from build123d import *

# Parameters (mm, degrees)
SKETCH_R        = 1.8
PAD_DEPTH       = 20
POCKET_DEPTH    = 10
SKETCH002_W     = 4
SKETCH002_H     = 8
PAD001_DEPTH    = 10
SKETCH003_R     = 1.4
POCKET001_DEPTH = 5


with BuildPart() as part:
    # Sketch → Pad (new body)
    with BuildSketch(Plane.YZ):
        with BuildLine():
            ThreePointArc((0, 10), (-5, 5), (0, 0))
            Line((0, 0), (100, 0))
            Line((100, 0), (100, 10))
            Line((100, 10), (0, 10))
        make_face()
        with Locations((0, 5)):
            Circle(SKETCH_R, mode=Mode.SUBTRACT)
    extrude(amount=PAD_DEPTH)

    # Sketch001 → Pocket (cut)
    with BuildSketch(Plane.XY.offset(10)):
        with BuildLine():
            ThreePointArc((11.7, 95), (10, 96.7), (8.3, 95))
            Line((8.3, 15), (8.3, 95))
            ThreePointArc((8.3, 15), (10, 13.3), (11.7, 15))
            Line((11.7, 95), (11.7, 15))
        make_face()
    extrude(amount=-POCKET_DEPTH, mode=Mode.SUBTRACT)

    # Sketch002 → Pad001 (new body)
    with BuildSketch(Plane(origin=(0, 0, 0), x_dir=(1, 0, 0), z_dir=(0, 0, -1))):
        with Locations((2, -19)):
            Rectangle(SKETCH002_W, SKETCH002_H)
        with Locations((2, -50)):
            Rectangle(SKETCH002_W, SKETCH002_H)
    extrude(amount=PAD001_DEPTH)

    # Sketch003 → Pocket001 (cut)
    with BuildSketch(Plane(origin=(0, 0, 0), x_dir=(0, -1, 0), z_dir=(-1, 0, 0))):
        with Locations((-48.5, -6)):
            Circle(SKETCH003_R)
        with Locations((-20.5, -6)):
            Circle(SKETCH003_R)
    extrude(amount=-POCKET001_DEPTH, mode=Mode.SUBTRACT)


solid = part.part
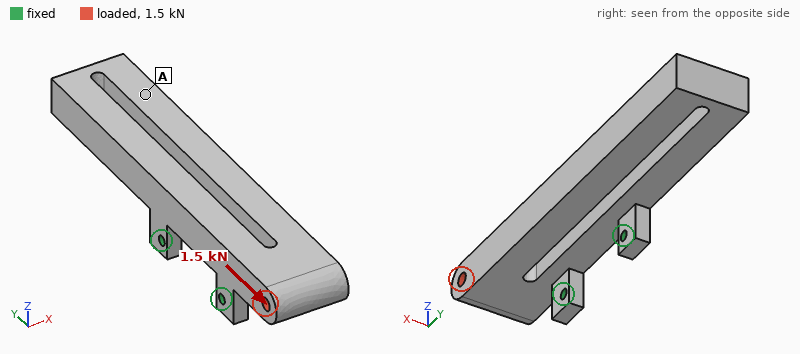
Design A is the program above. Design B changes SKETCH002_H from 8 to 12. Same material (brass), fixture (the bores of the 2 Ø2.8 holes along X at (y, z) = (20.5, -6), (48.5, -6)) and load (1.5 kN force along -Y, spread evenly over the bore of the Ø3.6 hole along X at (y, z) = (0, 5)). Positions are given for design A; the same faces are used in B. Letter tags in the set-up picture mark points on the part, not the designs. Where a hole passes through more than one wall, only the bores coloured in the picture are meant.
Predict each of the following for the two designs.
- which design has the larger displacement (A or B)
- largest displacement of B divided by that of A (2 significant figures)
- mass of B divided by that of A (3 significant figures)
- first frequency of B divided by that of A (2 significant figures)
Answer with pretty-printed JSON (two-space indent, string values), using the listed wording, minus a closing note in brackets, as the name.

{
  "which design has the larger displacement": "A",
  "largest displacement of B divided by that of A": "0.90",
  "mass of B divided by that of A": "1.02",
  "first frequency of B divided by that of A": "1.1"
}
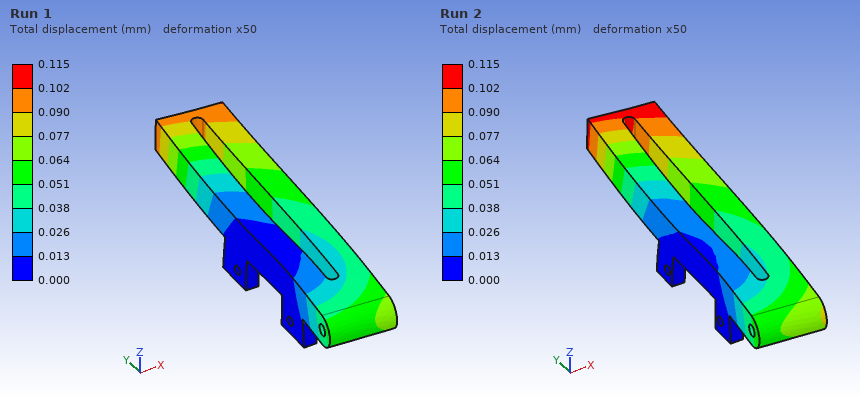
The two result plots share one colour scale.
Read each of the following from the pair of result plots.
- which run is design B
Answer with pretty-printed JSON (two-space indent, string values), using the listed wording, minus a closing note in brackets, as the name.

{
  "which run is design B": "Run 1"
}
